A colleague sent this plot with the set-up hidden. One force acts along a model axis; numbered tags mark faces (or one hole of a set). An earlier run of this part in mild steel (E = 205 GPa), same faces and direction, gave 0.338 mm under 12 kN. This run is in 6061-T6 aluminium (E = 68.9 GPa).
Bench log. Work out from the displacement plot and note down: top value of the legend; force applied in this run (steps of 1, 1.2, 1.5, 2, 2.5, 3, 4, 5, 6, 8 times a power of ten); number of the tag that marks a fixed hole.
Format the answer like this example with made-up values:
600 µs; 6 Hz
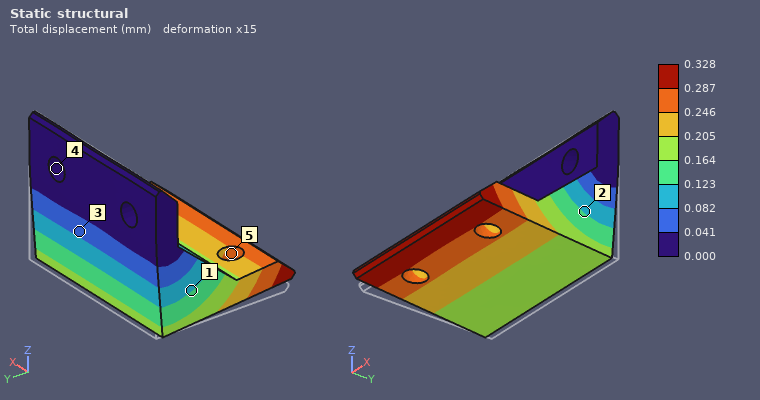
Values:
0.328 mm; 4 kN; 4
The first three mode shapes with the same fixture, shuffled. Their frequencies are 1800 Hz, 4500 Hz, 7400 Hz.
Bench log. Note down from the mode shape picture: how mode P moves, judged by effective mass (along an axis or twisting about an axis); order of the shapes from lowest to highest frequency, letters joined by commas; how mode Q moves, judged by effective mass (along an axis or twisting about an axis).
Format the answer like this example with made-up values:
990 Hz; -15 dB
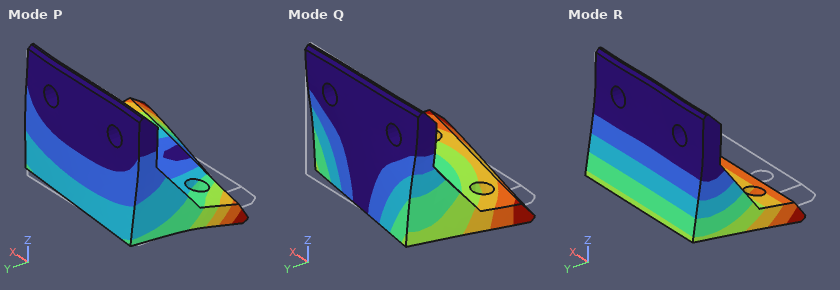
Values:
along X; R, Q, P; along X
